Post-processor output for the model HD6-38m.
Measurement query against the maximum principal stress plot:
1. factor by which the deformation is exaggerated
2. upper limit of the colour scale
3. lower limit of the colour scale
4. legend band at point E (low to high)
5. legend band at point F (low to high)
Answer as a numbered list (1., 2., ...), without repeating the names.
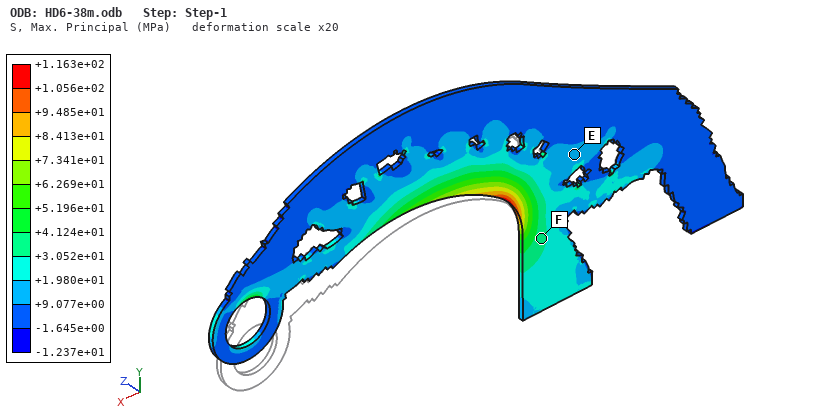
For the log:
1. 20
2. +1.163e+02 MPa
3. -1.237e+01 MPa
4. +9.077e+00 to +1.980e+01 MPa
5. +3.052e+01 to +4.124e+01 MPa
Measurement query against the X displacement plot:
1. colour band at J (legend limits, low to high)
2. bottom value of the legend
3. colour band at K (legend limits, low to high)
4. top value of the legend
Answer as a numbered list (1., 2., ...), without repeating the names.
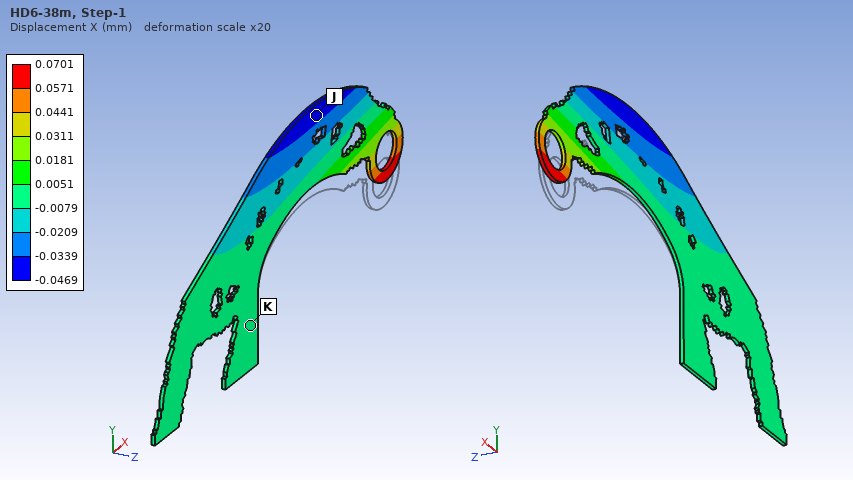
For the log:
1. -0.0469 to -0.0339 mm
2. -0.0469 mm
3. -0.0079 to 0.0051 mm
4. 0.0701 mm
